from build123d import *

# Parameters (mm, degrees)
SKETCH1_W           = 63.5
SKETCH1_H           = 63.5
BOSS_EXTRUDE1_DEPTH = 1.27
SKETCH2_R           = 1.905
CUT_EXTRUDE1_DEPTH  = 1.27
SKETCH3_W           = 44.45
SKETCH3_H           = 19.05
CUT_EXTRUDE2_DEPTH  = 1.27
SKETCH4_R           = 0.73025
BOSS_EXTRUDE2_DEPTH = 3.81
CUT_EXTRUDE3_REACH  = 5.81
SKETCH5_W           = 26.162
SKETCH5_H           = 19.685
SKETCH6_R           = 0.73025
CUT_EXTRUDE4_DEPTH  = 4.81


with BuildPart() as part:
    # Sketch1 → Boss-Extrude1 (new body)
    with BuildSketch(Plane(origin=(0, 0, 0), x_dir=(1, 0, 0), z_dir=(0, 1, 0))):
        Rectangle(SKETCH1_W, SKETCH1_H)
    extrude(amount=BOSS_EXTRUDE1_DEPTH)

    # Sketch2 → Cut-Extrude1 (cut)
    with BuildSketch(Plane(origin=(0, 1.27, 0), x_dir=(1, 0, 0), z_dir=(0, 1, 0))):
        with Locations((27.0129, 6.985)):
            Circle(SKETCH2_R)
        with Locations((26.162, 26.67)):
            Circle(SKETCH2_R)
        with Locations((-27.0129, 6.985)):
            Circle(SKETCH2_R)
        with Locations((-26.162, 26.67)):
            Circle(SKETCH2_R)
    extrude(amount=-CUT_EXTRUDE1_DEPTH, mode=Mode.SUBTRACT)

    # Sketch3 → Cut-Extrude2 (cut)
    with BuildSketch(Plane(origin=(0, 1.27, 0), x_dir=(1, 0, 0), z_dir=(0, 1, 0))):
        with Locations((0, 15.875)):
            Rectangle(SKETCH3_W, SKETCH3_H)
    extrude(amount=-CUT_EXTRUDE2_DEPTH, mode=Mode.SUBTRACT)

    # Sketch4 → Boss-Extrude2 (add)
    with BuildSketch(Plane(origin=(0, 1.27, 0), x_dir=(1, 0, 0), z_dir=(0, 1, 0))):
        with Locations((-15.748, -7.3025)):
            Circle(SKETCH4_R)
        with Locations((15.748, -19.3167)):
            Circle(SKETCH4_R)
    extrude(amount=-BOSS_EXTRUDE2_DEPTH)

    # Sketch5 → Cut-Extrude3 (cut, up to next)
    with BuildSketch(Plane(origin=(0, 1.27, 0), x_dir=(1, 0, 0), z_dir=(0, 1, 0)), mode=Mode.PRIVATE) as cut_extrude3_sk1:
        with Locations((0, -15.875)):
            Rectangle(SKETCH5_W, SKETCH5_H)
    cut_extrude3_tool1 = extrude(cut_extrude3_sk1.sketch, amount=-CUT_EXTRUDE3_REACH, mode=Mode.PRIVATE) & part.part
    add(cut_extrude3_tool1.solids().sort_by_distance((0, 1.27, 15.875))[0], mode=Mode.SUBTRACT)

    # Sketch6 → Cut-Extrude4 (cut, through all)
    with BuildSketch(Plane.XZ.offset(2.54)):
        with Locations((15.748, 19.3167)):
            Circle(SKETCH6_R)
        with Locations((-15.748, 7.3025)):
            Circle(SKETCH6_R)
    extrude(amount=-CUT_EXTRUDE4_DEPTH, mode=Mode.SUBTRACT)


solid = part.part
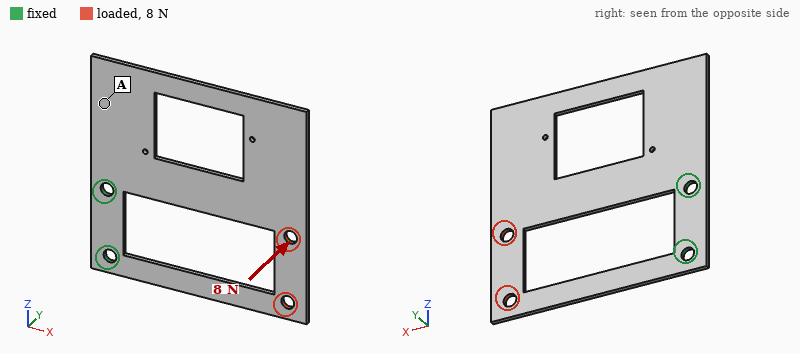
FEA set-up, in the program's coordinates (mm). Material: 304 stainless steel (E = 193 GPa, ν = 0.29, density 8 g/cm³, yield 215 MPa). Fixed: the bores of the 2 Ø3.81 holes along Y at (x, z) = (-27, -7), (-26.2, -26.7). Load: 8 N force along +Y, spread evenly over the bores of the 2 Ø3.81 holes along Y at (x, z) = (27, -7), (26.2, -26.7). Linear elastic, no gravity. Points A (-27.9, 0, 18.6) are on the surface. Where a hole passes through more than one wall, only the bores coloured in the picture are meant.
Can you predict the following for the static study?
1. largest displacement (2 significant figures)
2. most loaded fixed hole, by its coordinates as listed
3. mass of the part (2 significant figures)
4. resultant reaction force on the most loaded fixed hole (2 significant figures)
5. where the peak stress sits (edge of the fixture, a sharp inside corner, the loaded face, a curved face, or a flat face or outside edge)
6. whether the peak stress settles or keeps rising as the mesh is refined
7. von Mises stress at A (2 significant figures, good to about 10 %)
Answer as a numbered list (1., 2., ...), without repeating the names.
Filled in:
1. 0.65 mm
2. (-27, -7)
3. 27 g
4. 4.8 N
5. edge of the fixture
6. keeps rising
7. 11 MPa
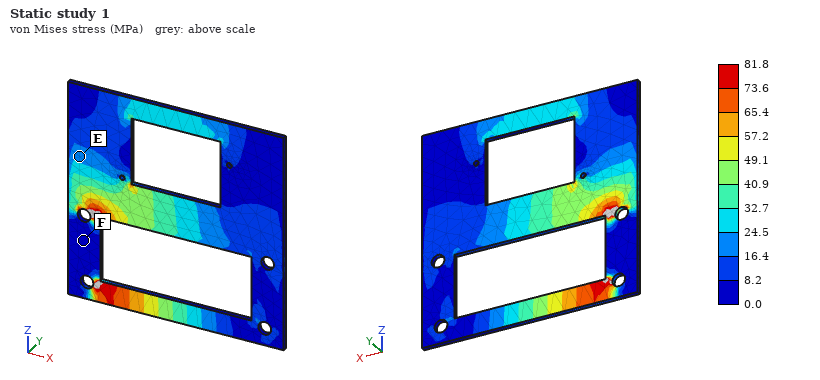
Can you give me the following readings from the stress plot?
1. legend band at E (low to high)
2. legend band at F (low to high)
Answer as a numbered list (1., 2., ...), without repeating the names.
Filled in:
1. 16.4 to 24.5 MPa
2. 0.0 to 8.2 MPa
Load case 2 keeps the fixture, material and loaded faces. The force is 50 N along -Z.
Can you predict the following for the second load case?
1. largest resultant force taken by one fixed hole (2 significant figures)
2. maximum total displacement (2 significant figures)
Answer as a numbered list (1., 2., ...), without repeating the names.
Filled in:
1. 79 N
2. 42 µm
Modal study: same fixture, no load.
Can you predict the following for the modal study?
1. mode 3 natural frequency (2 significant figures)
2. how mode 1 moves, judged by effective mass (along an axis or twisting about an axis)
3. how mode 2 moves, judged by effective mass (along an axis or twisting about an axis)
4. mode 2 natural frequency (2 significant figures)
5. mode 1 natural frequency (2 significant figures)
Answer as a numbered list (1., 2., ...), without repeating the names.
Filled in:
1. 840 Hz
2. along Y
3. twisting about X
4. 410 Hz
5. 190 Hz
